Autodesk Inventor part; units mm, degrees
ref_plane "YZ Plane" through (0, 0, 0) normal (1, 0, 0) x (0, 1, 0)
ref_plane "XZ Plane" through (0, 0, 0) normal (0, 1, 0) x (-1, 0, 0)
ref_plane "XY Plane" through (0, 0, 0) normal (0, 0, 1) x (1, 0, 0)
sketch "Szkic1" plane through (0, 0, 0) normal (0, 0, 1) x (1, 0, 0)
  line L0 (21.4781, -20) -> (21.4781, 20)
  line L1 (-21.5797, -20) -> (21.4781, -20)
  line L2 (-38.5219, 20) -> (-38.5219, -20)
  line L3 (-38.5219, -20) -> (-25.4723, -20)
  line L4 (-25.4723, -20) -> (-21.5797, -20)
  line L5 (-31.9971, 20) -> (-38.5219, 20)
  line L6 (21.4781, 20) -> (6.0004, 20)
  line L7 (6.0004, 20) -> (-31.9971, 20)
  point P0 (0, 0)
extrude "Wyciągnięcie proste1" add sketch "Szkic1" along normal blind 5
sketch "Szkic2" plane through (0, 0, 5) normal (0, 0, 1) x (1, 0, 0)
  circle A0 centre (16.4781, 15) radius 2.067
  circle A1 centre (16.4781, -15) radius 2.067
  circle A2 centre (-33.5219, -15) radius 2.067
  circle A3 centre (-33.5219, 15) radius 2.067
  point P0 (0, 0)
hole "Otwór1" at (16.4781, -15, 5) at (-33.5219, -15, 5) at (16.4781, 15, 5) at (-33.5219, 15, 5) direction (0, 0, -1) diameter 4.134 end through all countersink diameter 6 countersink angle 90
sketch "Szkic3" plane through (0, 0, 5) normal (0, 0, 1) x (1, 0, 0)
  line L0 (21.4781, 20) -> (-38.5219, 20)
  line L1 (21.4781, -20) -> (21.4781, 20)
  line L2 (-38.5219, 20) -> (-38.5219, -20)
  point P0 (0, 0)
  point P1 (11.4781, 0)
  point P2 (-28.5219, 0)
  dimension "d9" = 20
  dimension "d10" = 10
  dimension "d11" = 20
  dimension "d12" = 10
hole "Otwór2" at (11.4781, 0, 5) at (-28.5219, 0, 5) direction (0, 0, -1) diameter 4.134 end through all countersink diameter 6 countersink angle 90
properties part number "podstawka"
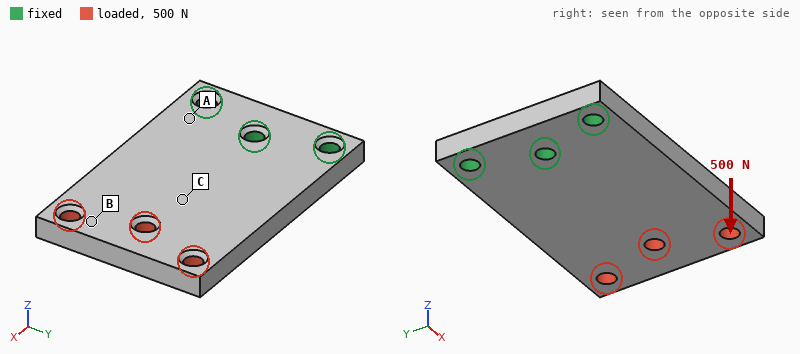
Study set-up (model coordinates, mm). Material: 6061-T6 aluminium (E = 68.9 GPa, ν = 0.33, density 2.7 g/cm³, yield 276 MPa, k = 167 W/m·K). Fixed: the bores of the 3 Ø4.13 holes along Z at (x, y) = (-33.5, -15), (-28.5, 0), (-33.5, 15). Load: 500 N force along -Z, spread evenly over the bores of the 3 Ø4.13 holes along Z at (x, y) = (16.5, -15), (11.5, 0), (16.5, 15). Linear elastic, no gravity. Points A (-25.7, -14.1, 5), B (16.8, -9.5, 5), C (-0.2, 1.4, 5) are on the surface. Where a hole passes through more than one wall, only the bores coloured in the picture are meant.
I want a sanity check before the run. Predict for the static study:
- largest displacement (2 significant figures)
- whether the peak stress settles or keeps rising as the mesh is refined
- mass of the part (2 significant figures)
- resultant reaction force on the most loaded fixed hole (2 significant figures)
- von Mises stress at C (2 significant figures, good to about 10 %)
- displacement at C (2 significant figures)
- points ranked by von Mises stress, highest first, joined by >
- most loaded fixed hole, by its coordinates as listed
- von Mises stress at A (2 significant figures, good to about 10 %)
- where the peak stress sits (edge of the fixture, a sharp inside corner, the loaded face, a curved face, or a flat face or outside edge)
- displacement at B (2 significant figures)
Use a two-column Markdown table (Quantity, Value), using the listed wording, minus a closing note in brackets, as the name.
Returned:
| Quantity | Value |
|---|---|
| largest displacement | 0.64 mm |
| whether the peak stress settles or keeps rising as the mesh is refined | keeps rising |
| mass of the part | 31 g |
| resultant reaction force on the most loaded fixed hole | 1.0 kN |
| von Mises stress at C | 40 MPa |
| displacement at C | 0.28 mm |
| points ranked by von Mises stress, highest first, joined by > | A > C > B |
| most loaded fixed hole, by its coordinates as listed | (-28.5, 0) |
| von Mises stress at A | 91 MPa |
| where the peak stress sits | edge of the fixture |
| displacement at B | 0.56 mm |
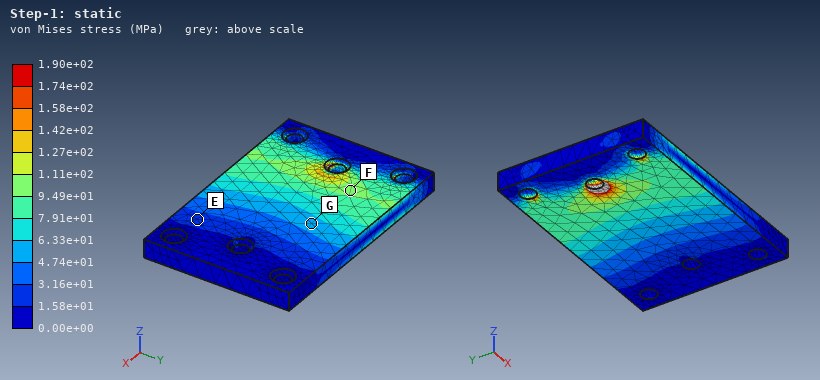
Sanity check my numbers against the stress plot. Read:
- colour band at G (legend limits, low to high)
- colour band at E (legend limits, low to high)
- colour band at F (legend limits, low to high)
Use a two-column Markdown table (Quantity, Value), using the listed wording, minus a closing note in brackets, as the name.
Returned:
| Quantity | Value |
|---|---|
| colour band at G | 4.74e+01 to 6.33e+01 MPa |
| colour band at E | 1.58e+01 to 3.16e+01 MPa |
| colour band at F | 9.49e+01 to 1.11e+02 MPa |
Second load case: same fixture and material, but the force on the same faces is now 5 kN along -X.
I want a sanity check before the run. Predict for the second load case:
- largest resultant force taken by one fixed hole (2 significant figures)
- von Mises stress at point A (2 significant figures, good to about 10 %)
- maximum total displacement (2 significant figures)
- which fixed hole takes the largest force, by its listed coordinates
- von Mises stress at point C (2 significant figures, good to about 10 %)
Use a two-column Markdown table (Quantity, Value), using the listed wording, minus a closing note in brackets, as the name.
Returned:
| Quantity | Value |
|---|---|
| largest resultant force taken by one fixed hole | 2.1 kN |
| von Mises stress at point A | 16 MPa |
| maximum total displacement | 0.10 mm |
| which fixed hole takes the largest force, by its listed coordinates | (-28.5, 0) |
| von Mises stress at point C | 13 MPa |
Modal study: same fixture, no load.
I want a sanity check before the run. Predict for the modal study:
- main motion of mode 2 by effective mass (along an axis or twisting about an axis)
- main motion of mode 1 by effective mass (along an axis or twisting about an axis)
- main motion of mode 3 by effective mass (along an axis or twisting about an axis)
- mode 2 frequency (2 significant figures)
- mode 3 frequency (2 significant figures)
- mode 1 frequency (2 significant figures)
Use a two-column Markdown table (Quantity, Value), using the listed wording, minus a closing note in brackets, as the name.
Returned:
| Quantity | Value |
|---|---|
| main motion of mode 2 by effective mass | twisting about X |
| main motion of mode 1 by effective mass | along Z |
| main motion of mode 3 by effective mass | along Y |
| mode 2 frequency | 4200 Hz |
| mode 3 frequency | 8400 Hz |
| mode 1 frequency | 1600 Hz |
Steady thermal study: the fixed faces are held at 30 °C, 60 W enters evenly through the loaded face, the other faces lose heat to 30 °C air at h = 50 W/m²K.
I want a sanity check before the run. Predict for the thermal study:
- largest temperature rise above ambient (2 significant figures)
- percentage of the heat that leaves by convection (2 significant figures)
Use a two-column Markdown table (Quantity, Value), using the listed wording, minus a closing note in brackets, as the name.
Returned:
| Quantity | Value |
|---|---|
| largest temperature rise above ambient | 80 K |
| percentage of the heat that leaves by convection | 17 % |
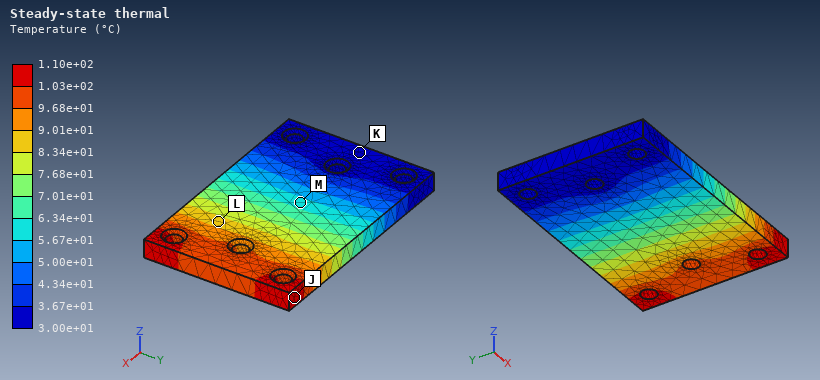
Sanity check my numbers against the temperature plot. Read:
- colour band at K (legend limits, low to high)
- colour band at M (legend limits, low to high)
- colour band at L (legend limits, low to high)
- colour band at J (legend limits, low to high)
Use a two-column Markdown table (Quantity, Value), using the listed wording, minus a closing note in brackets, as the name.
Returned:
| Quantity | Value |
|---|---|
| colour band at K | 3.00e+01 to 3.67e+01 °C |
| colour band at M | 5.67e+01 to 6.34e+01 °C |
| colour band at L | 8.34e+01 to 9.01e+01 °C |
| colour band at J | 1.03e+02 to 1.10e+02 °C |
